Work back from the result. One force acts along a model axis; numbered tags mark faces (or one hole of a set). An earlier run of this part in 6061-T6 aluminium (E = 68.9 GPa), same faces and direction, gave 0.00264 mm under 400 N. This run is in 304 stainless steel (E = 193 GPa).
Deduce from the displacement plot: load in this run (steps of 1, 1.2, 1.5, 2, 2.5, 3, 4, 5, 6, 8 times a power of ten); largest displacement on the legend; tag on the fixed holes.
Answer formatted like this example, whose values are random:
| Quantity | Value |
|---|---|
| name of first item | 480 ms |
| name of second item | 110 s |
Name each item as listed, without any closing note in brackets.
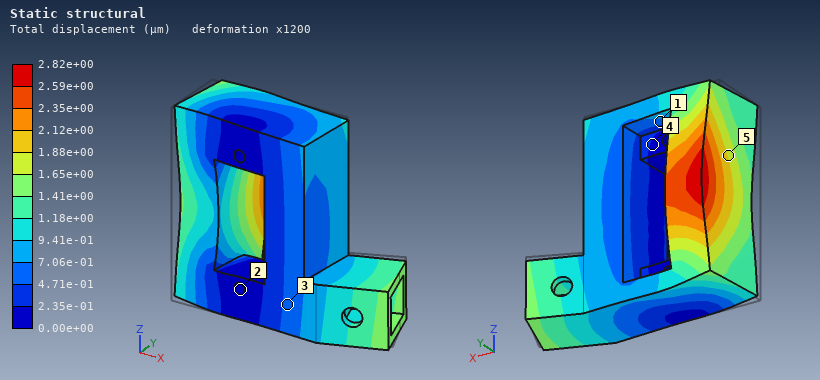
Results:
| Quantity | Value |
|---|---|
| load in this run | 1.2 kN |
| largest displacement on the legend | 2.82e+00 µm |
| tag on the fixed holes | 2 |
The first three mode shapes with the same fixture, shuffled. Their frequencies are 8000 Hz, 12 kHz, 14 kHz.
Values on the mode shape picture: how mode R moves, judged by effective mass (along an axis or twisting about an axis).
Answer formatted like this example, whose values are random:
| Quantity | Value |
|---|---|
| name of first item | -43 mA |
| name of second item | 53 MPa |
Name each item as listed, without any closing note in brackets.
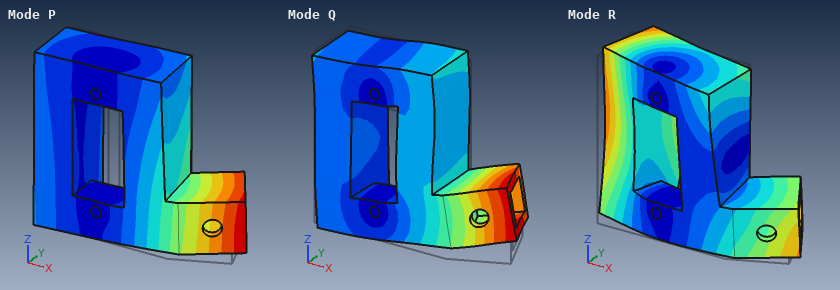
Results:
| Quantity | Value |
|---|---|
| how mode R moves, judged by effective mass | along Y |
